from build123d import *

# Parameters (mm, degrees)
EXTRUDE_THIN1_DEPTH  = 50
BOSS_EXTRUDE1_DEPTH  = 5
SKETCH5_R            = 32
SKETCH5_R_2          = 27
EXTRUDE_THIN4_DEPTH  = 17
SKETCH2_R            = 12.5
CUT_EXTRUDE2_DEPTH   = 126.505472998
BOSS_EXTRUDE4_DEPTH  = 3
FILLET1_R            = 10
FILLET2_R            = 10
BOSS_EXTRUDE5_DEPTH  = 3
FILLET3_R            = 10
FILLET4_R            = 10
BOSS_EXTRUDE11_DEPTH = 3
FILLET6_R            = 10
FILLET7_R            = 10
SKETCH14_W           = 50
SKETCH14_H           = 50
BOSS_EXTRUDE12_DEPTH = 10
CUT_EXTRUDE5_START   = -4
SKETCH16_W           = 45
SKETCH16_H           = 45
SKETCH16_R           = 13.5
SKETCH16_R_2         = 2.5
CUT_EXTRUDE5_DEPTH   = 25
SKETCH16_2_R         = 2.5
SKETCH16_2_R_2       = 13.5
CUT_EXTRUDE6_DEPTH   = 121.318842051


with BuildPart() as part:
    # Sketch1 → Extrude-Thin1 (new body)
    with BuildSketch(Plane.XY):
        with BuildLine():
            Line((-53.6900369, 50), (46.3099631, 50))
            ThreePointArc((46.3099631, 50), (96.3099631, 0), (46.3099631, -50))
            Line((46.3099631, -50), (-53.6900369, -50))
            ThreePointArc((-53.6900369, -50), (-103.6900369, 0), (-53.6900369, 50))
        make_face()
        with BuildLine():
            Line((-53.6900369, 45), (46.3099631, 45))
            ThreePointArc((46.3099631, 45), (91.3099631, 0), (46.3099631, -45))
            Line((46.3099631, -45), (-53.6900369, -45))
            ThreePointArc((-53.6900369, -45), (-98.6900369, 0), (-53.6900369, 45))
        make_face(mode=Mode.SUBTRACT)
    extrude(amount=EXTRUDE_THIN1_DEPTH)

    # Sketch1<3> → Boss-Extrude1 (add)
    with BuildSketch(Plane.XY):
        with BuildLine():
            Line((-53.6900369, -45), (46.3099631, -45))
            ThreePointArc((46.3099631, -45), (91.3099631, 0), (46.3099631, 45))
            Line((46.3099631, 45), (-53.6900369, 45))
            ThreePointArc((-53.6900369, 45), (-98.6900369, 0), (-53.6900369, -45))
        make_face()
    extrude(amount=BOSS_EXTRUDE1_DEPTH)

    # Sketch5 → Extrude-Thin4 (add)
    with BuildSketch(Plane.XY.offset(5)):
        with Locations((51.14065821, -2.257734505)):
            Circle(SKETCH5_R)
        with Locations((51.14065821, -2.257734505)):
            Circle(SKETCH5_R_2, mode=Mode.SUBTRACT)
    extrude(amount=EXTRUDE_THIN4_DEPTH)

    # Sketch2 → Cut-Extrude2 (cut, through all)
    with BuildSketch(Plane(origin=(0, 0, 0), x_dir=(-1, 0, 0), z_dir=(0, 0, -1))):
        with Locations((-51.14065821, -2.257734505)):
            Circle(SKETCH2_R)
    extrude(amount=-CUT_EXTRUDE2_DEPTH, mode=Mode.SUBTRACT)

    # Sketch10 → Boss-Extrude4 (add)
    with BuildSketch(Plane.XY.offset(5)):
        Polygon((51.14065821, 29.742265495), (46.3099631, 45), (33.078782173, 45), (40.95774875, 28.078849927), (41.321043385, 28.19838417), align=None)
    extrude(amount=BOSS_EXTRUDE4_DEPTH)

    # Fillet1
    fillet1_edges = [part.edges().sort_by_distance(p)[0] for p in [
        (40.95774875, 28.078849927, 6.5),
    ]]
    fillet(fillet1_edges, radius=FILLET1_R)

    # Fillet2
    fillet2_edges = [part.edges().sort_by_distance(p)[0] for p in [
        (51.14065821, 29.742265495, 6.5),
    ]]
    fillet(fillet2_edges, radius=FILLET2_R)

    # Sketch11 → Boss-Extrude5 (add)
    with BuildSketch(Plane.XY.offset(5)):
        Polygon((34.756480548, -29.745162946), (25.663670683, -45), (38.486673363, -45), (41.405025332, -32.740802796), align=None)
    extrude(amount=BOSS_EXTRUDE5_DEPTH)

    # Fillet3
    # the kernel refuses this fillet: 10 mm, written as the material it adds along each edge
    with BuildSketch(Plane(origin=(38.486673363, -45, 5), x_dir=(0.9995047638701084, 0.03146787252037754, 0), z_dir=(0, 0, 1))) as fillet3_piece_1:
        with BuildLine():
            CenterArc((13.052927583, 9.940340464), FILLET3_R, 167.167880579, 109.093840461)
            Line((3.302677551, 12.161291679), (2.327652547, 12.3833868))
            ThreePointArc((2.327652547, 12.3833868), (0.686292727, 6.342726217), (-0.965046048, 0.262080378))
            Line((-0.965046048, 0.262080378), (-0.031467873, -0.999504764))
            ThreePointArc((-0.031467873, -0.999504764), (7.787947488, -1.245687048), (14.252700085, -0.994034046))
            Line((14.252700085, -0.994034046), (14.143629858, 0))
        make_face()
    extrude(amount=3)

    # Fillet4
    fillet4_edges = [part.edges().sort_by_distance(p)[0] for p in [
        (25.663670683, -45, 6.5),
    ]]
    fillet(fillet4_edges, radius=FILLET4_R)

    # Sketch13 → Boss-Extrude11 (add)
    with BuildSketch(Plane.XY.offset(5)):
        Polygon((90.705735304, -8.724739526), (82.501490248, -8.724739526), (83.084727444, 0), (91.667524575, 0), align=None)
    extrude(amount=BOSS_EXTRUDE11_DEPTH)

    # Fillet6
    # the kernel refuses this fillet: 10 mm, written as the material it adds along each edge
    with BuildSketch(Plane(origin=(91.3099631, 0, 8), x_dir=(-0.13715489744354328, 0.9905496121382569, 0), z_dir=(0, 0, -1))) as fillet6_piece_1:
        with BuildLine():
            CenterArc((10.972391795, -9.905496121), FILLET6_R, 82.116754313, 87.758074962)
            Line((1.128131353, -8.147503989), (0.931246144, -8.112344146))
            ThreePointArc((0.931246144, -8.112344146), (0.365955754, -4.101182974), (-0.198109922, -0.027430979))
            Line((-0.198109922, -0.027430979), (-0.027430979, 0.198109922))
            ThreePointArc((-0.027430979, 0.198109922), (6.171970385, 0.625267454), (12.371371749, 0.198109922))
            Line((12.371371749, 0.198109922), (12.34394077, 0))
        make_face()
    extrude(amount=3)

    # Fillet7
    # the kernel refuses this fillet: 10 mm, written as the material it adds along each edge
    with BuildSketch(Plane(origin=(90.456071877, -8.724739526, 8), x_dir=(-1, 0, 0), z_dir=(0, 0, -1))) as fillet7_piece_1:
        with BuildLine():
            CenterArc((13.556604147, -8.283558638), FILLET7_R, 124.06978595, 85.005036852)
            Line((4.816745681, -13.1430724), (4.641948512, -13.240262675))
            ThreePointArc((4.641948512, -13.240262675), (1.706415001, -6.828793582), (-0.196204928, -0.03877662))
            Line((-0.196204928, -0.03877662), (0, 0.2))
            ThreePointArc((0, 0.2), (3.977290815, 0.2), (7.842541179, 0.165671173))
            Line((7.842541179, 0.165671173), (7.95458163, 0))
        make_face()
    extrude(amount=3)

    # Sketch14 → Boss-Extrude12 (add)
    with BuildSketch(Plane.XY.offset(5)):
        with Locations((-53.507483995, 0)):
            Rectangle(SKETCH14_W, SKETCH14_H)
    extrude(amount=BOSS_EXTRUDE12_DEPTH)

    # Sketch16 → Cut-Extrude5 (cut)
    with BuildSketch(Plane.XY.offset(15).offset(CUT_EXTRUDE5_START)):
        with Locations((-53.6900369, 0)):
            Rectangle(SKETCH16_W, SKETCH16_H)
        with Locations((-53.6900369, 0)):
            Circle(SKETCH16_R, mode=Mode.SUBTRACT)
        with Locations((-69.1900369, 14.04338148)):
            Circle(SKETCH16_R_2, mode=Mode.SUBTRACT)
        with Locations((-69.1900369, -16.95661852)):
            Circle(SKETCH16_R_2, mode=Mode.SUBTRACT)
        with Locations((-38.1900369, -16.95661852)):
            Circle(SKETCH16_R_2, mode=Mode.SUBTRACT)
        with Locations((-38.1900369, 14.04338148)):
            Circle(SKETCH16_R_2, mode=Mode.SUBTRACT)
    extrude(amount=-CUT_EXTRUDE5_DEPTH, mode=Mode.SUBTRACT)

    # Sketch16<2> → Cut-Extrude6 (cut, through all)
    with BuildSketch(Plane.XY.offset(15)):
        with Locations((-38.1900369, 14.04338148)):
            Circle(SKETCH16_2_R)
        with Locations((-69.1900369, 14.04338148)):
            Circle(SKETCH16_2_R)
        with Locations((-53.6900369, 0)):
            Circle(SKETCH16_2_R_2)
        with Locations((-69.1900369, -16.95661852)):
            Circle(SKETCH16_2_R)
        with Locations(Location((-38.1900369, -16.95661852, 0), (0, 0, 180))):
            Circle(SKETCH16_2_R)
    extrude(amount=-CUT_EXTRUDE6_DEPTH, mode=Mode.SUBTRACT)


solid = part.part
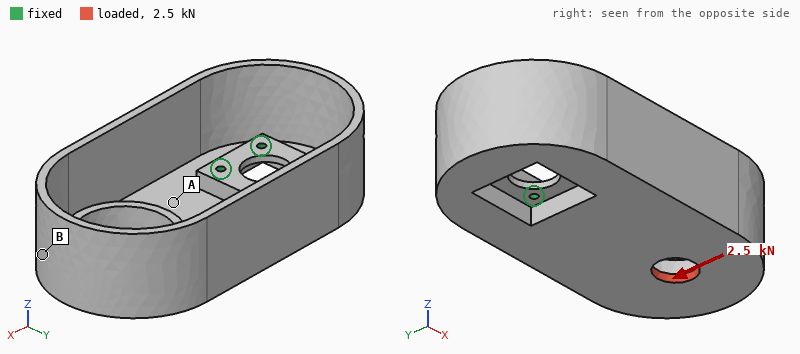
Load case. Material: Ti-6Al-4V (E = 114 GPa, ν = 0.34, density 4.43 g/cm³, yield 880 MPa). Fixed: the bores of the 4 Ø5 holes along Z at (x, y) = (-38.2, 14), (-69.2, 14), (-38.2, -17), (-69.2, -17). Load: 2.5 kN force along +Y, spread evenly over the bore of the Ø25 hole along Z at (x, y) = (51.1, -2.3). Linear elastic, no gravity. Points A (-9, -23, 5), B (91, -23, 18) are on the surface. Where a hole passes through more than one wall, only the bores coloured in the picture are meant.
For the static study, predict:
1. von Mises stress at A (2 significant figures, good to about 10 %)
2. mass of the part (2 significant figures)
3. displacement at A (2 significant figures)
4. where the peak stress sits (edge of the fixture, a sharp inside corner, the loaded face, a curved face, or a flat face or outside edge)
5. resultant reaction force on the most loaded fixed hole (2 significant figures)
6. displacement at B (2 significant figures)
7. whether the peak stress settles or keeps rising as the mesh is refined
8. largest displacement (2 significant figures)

13 MPa
960 g
28 µm
edge of the fixture
3.5 kN
93 µm
keeps rising
95 µm
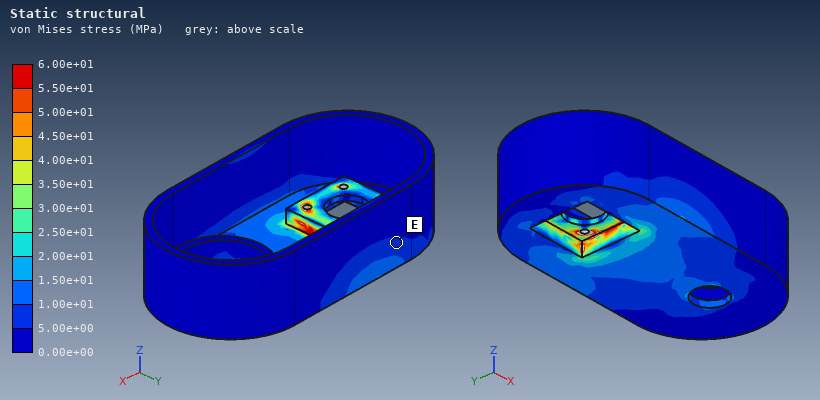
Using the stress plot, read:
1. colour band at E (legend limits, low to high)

5.00e+00 to 1.00e+01 MPa
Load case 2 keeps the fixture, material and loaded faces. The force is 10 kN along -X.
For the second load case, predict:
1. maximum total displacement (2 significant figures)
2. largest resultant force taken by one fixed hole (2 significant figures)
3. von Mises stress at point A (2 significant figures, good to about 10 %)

0.19 mm
3.4 kN
28 MPa
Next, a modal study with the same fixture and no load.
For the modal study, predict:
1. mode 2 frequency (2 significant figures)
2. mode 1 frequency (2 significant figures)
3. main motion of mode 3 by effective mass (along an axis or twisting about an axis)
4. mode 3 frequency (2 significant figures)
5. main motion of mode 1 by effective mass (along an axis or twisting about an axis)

670 Hz
400 Hz
along Y
1300 Hz
along Z
